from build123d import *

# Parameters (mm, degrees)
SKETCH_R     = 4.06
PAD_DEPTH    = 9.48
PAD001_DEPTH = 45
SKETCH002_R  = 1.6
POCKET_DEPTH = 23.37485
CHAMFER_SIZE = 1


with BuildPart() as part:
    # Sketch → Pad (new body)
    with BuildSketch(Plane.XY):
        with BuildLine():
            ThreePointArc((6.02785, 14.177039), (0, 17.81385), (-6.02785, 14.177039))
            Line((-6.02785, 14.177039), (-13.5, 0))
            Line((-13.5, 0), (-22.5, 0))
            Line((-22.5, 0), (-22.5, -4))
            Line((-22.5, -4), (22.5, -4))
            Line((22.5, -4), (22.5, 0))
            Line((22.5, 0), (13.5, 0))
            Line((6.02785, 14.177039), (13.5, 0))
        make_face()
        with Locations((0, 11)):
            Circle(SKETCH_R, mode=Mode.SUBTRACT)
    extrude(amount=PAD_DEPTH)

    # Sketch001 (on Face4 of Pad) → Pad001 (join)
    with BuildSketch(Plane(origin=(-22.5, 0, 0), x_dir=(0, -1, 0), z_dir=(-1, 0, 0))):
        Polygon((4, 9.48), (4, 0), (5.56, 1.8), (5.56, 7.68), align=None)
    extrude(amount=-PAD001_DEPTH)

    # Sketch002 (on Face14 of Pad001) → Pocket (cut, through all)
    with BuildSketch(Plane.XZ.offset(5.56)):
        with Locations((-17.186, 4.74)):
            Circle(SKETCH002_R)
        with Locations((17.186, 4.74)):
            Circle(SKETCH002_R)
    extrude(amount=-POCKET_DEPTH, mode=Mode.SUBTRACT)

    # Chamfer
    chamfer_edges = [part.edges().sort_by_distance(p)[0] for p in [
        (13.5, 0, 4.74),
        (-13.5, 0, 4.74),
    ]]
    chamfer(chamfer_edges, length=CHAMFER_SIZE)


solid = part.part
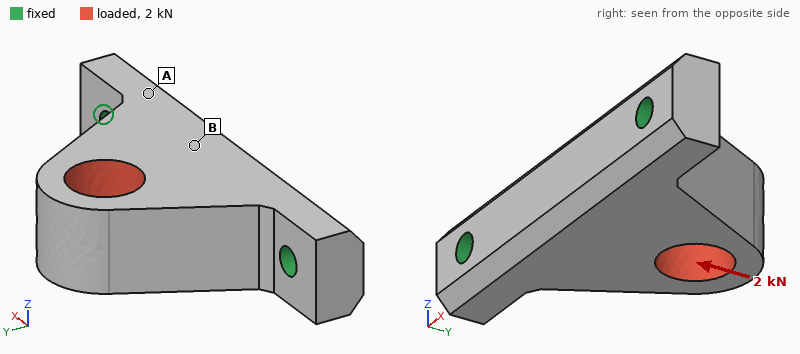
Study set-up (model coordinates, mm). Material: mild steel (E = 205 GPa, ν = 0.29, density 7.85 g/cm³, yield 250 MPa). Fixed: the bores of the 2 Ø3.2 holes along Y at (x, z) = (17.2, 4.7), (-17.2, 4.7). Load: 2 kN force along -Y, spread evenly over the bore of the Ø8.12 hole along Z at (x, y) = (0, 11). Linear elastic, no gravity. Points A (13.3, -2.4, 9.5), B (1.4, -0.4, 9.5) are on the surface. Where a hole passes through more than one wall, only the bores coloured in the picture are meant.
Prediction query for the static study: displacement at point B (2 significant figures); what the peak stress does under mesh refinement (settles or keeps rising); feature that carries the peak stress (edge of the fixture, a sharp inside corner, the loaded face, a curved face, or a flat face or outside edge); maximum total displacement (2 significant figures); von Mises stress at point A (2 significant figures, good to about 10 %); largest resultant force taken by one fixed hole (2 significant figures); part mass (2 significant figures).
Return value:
3.6 µm
keeps rising
edge of the fixture
4.3 µm
29 MPa
1.2 kN
36 g
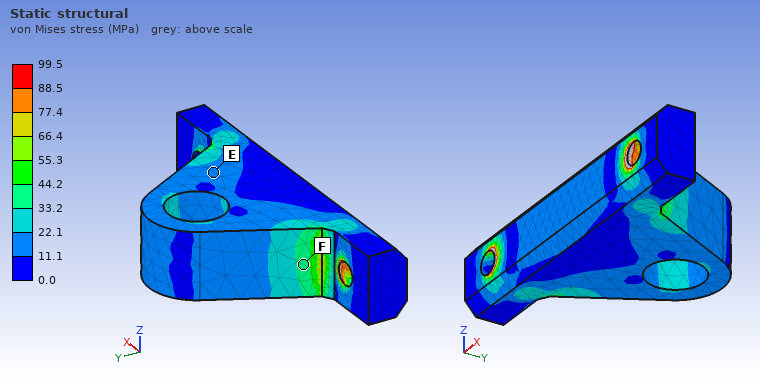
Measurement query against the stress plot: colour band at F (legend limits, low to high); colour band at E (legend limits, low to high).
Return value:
33.2 to 44.2 MPa
11.1 to 22.1 MPa
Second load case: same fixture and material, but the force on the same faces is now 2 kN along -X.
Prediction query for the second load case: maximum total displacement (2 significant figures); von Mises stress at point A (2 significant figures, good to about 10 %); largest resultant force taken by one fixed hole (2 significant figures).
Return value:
7.7 µm
22 MPa
1.4 kN
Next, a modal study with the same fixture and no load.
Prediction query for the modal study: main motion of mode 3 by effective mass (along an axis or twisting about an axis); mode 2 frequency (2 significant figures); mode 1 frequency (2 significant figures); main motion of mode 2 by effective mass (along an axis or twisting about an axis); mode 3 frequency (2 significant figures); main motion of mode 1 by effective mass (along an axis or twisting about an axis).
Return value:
along Z
23 kHz
9500 Hz
along Y
26 kHz
along Z
